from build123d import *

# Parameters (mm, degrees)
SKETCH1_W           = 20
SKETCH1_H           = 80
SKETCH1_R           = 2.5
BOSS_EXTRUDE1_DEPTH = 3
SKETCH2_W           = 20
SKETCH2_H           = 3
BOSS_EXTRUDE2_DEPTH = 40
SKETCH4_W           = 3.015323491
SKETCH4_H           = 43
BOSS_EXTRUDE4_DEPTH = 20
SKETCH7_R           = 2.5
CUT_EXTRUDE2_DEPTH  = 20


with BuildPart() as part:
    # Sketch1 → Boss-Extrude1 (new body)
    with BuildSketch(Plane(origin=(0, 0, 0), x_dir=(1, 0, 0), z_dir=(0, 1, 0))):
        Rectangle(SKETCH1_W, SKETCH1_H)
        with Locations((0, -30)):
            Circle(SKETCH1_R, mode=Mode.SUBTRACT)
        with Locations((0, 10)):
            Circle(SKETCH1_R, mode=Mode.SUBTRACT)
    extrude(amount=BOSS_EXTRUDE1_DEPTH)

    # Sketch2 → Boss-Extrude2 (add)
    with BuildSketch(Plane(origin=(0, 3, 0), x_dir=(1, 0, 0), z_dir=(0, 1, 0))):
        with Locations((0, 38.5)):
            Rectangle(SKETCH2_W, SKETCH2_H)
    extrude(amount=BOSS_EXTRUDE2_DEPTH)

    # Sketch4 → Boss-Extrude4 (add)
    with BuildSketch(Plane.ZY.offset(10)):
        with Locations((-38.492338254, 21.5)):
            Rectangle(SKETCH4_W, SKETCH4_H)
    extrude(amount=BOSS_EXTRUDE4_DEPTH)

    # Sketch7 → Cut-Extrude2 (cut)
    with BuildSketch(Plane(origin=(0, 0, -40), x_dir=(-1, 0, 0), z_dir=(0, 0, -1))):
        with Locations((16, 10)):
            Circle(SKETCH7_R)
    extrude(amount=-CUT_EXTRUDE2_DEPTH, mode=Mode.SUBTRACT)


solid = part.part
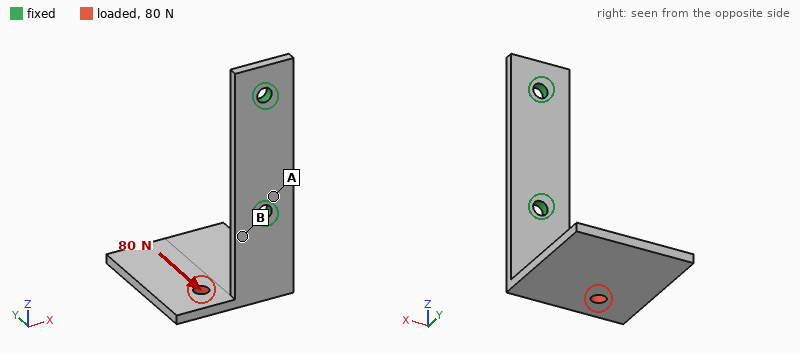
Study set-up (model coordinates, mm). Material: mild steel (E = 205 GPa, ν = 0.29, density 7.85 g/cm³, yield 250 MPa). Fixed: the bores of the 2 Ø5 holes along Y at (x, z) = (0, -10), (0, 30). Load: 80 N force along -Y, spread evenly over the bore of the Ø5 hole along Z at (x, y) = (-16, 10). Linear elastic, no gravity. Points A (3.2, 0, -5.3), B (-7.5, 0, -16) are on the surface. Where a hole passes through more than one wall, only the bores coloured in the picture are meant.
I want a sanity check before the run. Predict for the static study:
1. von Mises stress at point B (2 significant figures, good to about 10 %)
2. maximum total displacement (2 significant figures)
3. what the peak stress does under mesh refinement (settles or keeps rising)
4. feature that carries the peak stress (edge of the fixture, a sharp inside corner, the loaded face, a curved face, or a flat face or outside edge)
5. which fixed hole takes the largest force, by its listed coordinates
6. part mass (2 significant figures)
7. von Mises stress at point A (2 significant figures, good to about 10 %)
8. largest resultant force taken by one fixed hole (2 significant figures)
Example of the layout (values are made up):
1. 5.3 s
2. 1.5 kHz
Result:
1. 64 MPa
2. 0.22 mm
3. keeps rising
4. edge of the fixture
5. (0, -10)
6. 75 g
7. 13 MPa
8. 83 N
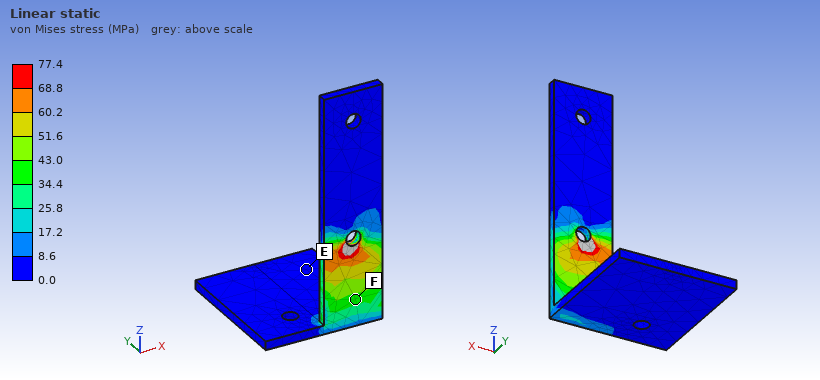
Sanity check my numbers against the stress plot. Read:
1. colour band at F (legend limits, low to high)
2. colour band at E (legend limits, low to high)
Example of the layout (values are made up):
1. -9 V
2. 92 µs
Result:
1. 34.4 to 43.0 MPa
2. 0.0 to 8.6 MPa
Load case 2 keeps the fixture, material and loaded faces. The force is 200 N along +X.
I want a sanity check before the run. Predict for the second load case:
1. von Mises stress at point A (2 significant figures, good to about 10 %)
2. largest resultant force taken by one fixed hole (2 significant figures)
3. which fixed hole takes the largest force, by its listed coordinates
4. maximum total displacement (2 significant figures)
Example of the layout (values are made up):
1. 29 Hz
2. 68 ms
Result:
1. 13 MPa
2. 290 N
3. (0, -10)
4. 0.16 mm
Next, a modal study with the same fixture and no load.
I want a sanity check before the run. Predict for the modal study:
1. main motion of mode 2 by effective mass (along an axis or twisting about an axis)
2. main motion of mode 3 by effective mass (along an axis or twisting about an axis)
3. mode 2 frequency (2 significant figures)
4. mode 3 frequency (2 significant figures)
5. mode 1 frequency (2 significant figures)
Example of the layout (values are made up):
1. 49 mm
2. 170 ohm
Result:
1. along X
2. along Y
3. 680 Hz
4. 1600 Hz
5. 480 Hz
